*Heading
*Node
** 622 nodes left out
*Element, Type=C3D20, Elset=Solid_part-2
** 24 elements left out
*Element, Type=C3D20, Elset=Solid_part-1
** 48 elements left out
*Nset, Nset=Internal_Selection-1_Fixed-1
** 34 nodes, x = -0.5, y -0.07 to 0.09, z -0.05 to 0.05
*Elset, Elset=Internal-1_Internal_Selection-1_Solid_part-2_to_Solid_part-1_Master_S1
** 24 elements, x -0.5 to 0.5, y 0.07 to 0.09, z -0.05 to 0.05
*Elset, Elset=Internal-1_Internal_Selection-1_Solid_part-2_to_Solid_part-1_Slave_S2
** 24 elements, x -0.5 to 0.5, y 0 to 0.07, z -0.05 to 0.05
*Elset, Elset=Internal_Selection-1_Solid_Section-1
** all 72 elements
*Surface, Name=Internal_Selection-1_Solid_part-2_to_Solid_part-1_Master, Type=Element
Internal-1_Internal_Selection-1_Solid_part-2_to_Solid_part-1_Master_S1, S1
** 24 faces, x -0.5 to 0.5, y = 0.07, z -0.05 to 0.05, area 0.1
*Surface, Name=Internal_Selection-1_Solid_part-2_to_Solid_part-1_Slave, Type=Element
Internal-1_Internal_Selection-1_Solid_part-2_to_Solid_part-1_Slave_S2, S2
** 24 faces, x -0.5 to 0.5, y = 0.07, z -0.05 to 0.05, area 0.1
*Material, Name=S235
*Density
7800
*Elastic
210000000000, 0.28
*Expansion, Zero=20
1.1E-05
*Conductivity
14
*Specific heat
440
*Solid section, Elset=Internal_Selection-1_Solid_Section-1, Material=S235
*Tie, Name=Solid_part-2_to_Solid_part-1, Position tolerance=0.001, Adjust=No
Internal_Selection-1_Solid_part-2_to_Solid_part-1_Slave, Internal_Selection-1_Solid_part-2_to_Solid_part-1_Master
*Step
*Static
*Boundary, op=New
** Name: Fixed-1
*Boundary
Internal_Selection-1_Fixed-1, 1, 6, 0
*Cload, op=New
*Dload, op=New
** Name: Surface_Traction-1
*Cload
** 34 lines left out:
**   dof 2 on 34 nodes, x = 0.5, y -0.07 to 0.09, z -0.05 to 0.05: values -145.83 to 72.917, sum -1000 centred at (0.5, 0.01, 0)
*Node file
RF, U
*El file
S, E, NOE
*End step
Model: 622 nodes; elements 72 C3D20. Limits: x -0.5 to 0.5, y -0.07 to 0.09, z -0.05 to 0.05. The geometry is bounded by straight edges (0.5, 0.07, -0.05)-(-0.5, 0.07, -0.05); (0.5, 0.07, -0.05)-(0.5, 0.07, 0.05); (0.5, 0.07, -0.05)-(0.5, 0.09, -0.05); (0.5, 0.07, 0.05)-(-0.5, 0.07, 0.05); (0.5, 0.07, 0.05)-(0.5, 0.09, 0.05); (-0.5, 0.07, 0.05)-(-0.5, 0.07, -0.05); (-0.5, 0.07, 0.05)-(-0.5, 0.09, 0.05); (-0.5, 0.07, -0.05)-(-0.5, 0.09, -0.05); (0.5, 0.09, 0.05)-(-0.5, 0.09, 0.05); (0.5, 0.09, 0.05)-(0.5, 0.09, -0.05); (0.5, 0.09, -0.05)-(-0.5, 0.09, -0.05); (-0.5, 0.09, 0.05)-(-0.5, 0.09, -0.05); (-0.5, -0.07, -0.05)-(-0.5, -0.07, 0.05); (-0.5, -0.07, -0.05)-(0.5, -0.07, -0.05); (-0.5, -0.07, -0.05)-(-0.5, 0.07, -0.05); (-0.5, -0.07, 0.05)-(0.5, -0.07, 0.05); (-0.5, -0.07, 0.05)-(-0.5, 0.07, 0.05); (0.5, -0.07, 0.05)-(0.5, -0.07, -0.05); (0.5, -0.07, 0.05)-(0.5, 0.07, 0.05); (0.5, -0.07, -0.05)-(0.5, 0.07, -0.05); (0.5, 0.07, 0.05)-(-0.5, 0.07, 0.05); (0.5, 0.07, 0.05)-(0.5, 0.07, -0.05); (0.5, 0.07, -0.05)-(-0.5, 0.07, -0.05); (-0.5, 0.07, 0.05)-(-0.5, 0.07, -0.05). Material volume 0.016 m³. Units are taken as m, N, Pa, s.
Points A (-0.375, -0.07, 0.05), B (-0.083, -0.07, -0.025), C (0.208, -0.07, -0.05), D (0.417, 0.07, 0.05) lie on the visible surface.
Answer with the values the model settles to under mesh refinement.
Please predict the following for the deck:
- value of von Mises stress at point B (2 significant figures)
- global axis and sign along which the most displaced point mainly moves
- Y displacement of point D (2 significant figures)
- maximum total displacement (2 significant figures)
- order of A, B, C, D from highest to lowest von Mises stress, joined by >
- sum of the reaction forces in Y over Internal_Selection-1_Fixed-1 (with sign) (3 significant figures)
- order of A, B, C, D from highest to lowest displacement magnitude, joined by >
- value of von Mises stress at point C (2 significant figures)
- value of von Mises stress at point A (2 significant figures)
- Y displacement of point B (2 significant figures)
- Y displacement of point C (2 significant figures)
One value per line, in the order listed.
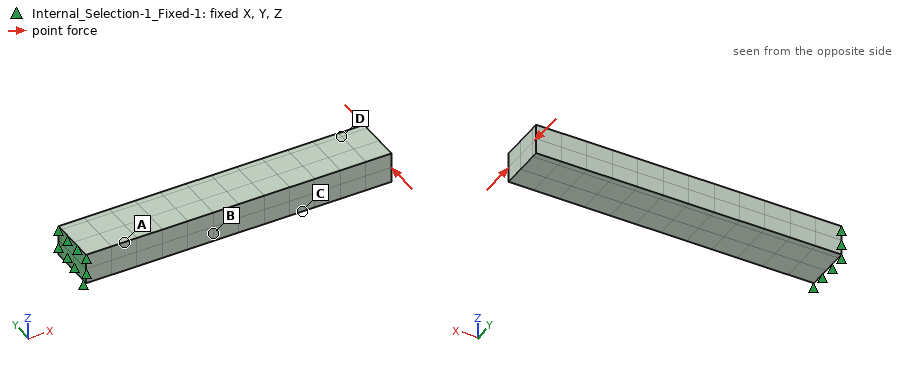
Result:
1.4e+06 Pa
-Y
-4.1e-05 m
4.7e-05 m
A > B > C > D
1000 N
D > C > B > A
6.8e+05 Pa
2.1e+06 Pa
-1.1e-05 m
-2.7e-05 m
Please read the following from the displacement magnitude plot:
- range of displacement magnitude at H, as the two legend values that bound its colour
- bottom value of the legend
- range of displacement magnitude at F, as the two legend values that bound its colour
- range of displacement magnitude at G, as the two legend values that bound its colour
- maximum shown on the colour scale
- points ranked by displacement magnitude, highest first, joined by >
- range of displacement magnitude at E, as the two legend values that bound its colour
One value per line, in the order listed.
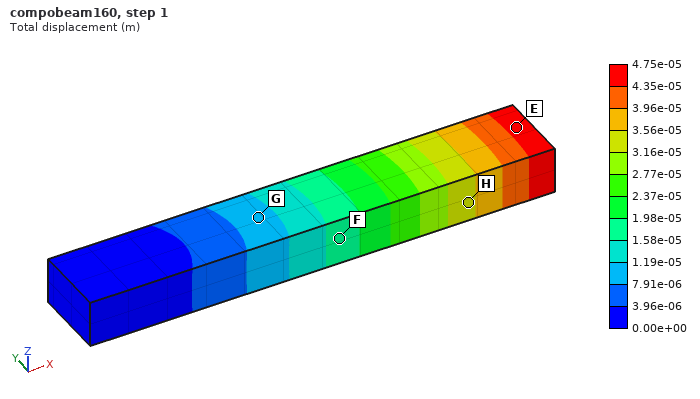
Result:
3.16e-05 to 3.56e-05 m
0.00e+00 m
1.58e-05 to 1.98e-05 m
7.91e-06 to 1.19e-05 m
4.75e-05 m
E > H > F > G
4.35e-05 to 4.75e-05 m
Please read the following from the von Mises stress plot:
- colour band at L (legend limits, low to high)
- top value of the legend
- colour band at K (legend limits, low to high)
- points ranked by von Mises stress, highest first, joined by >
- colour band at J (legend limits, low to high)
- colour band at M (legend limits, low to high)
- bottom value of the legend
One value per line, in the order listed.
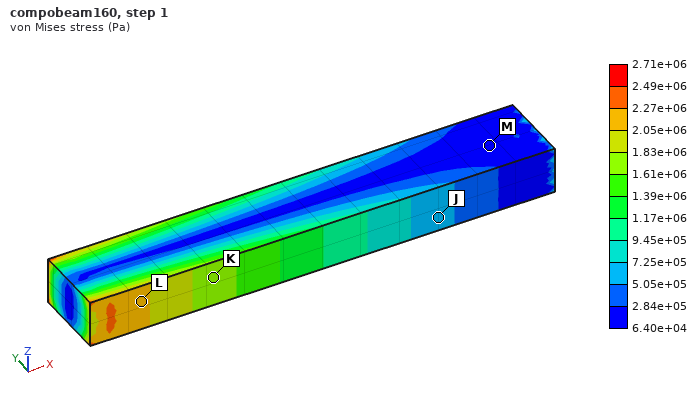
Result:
2.05e+06 to 2.27e+06 Pa
2.71e+06 Pa
1.61e+06 to 1.83e+06 Pa
L > K > J > M
5.05e+05 to 7.25e+05 Pa
6.40e+04 to 2.84e+05 Pa
6.40e+04 Pa
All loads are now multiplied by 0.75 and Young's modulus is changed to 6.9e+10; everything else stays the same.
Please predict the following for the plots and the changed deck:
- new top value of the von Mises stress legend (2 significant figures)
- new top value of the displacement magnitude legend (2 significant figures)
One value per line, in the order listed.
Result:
2.0e+06 Pa
1.1e-04 m
